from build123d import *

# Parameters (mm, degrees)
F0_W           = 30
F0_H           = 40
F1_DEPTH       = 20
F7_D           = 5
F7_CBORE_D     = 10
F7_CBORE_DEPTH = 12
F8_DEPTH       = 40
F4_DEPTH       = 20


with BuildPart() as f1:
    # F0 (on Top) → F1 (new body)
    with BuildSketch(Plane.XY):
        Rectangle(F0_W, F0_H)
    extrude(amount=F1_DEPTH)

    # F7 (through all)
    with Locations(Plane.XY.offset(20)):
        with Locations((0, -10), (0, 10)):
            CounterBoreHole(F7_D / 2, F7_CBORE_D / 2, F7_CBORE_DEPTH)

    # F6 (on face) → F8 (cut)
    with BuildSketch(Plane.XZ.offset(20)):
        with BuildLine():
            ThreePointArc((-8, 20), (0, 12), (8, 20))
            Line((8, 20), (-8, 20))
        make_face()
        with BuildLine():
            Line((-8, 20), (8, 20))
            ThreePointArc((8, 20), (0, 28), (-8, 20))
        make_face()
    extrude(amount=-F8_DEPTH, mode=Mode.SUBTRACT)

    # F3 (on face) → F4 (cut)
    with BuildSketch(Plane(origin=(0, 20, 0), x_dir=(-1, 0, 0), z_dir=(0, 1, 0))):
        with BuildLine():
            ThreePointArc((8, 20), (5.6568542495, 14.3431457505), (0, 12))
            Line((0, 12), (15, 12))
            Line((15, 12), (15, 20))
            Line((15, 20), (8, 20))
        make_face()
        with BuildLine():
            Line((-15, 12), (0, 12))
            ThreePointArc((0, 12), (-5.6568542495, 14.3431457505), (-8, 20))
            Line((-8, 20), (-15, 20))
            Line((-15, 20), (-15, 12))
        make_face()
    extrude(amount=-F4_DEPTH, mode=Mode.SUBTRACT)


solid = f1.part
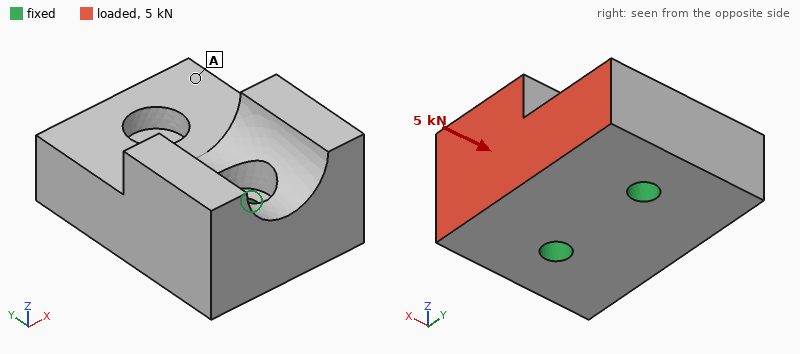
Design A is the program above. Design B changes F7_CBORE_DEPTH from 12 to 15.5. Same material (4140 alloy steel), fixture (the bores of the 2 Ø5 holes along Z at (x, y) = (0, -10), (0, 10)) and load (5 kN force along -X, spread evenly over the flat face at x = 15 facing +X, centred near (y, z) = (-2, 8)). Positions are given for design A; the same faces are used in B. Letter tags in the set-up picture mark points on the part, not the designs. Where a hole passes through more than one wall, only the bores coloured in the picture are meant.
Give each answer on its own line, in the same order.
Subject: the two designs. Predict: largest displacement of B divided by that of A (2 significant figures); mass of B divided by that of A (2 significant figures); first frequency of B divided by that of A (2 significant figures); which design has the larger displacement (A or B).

2.8
0.97
0.55
B
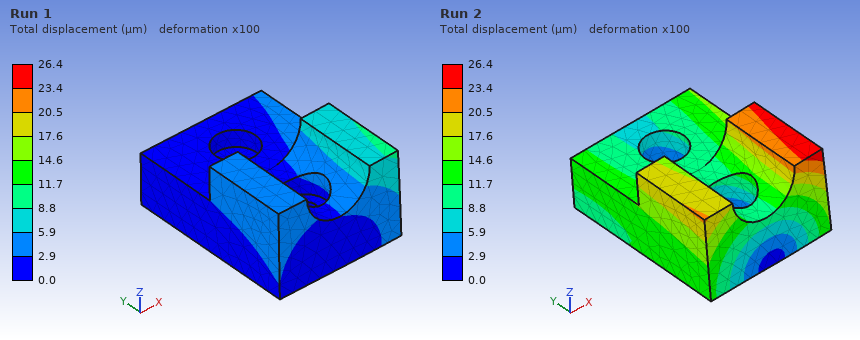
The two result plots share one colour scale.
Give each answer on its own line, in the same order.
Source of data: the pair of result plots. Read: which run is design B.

Run 2
